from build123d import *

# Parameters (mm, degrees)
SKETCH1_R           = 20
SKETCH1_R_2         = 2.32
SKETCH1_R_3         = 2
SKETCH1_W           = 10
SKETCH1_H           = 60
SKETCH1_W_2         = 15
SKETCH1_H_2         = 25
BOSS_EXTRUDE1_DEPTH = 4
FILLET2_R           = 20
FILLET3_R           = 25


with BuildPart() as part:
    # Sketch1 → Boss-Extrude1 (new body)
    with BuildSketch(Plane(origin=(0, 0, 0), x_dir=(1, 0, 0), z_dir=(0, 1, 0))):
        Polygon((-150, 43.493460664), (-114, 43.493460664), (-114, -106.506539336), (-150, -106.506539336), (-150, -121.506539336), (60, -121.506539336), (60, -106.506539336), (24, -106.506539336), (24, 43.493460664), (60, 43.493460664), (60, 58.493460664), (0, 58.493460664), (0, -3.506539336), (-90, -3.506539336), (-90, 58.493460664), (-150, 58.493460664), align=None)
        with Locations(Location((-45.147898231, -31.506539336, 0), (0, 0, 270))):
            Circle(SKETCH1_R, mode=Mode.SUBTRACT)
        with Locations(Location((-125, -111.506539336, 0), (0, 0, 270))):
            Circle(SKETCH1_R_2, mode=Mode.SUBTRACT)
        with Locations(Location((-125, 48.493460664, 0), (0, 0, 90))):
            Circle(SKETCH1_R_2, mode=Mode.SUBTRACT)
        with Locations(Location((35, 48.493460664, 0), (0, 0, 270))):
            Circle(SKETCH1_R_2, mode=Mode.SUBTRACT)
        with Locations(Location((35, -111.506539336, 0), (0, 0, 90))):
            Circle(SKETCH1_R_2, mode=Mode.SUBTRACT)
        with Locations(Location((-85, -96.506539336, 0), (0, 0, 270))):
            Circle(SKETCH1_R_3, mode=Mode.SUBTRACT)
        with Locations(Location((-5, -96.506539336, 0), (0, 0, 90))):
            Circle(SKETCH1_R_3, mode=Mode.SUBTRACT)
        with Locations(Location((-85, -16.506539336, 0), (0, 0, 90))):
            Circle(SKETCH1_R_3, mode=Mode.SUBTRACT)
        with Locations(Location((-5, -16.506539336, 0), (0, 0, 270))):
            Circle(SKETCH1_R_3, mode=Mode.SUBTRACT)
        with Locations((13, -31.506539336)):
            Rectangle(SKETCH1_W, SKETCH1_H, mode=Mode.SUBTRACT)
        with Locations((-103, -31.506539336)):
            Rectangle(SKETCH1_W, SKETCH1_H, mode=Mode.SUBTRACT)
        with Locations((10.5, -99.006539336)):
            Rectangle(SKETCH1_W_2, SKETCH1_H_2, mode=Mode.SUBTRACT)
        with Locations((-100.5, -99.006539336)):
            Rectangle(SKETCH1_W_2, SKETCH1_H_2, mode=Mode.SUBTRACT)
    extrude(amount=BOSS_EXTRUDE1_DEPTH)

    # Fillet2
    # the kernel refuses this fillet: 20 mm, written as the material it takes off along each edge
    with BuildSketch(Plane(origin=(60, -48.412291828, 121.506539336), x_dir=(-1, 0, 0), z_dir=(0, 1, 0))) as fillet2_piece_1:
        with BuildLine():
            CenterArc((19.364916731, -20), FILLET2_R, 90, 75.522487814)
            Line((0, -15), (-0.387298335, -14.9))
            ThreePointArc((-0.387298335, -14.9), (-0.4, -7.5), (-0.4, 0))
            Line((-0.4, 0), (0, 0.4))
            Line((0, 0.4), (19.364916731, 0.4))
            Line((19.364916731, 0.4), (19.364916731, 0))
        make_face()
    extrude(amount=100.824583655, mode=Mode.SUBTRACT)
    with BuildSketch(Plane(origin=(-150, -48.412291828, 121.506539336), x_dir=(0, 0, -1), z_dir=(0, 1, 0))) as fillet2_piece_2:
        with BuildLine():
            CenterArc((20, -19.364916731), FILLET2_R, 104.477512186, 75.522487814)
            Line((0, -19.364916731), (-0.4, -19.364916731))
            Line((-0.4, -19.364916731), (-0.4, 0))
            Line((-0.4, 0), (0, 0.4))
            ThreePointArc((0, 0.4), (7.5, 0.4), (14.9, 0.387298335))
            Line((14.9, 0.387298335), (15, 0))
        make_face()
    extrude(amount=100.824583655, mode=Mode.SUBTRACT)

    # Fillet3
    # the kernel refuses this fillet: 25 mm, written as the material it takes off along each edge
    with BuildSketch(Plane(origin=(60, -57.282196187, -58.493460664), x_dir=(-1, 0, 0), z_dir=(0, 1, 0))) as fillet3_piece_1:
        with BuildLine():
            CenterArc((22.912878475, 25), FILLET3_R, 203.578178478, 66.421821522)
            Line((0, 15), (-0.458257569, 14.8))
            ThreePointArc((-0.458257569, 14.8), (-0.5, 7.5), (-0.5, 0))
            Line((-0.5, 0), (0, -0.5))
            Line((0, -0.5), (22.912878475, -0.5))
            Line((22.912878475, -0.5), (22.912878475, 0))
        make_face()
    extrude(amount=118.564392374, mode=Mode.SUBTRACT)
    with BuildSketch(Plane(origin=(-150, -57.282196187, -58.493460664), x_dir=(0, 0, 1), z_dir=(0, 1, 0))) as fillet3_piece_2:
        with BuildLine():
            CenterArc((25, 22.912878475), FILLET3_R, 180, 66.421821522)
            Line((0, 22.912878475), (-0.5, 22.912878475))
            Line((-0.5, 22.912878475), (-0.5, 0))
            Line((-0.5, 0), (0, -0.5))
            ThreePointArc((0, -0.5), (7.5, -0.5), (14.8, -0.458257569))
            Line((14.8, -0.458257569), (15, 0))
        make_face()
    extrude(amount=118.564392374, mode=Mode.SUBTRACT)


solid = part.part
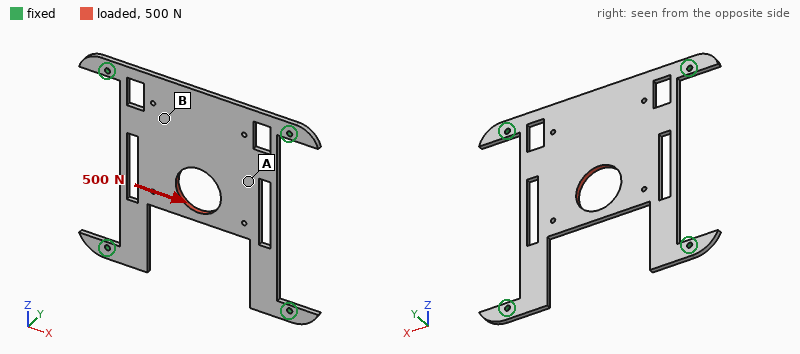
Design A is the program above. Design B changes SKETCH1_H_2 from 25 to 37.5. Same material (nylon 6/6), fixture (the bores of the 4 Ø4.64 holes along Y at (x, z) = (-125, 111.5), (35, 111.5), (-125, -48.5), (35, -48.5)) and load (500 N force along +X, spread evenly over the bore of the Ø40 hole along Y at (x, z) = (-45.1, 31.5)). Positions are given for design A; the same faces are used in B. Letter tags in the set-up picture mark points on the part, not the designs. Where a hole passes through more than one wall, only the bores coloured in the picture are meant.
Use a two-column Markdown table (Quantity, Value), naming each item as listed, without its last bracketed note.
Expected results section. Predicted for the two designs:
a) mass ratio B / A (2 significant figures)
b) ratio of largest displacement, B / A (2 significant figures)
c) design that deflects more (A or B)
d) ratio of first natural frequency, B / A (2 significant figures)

| Quantity | Value |
|---|---|
| mass ratio B / A | 0.98 |
| ratio of largest displacement, B / A | 1.3 |
| design that deflects more | B |
| ratio of first natural frequency, B / A | 0.97 |
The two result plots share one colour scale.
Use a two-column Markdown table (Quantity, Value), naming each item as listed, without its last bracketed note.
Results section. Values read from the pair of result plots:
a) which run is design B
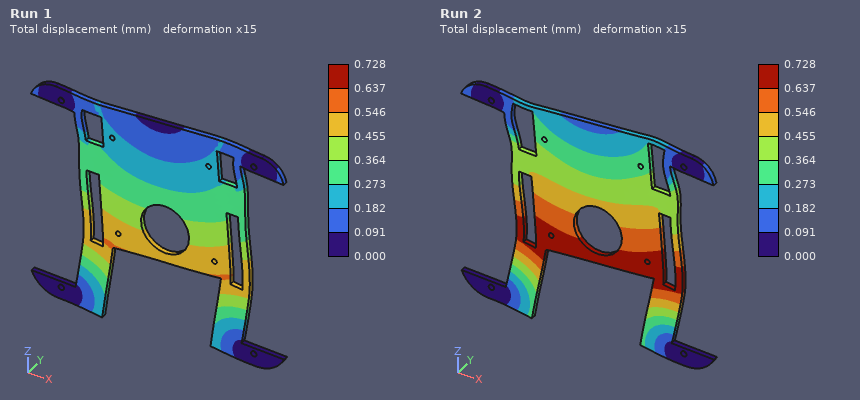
| Quantity | Value |
|---|---|
| which run is design B | Run 2 |
